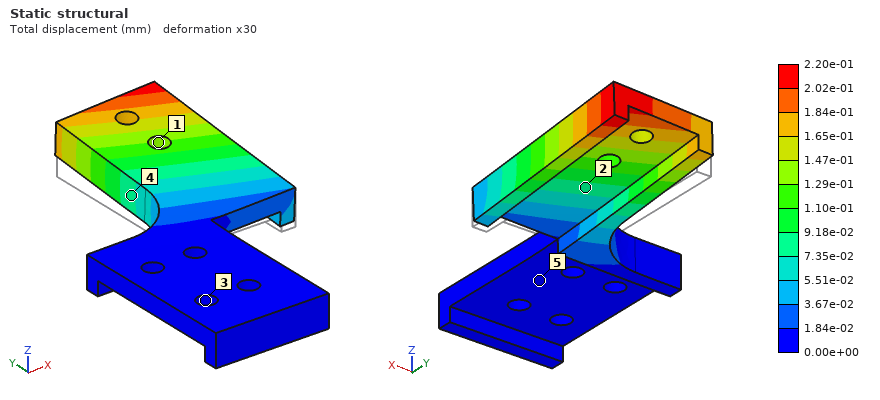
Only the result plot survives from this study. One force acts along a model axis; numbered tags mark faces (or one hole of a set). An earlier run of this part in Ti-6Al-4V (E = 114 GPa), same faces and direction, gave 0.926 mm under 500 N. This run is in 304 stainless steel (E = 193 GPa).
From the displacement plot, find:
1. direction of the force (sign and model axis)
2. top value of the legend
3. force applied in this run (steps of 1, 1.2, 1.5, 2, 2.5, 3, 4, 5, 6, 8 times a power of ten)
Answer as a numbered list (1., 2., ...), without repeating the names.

1. +Z
2. 2.20e-01 mm
3. 200 N
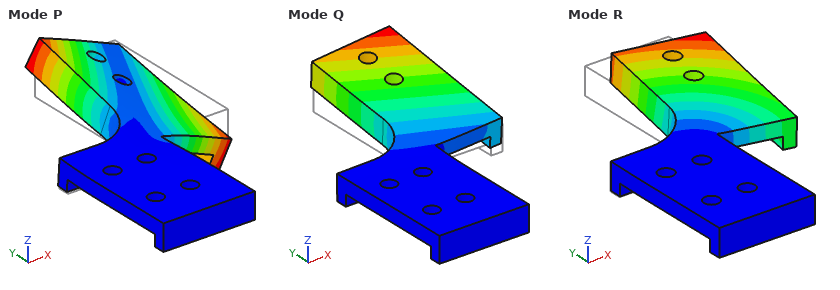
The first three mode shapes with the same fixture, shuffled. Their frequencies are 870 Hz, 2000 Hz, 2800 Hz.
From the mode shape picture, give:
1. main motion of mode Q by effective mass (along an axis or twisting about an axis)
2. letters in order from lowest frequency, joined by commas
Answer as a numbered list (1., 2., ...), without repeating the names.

1. along Z
2. Q, R, P
